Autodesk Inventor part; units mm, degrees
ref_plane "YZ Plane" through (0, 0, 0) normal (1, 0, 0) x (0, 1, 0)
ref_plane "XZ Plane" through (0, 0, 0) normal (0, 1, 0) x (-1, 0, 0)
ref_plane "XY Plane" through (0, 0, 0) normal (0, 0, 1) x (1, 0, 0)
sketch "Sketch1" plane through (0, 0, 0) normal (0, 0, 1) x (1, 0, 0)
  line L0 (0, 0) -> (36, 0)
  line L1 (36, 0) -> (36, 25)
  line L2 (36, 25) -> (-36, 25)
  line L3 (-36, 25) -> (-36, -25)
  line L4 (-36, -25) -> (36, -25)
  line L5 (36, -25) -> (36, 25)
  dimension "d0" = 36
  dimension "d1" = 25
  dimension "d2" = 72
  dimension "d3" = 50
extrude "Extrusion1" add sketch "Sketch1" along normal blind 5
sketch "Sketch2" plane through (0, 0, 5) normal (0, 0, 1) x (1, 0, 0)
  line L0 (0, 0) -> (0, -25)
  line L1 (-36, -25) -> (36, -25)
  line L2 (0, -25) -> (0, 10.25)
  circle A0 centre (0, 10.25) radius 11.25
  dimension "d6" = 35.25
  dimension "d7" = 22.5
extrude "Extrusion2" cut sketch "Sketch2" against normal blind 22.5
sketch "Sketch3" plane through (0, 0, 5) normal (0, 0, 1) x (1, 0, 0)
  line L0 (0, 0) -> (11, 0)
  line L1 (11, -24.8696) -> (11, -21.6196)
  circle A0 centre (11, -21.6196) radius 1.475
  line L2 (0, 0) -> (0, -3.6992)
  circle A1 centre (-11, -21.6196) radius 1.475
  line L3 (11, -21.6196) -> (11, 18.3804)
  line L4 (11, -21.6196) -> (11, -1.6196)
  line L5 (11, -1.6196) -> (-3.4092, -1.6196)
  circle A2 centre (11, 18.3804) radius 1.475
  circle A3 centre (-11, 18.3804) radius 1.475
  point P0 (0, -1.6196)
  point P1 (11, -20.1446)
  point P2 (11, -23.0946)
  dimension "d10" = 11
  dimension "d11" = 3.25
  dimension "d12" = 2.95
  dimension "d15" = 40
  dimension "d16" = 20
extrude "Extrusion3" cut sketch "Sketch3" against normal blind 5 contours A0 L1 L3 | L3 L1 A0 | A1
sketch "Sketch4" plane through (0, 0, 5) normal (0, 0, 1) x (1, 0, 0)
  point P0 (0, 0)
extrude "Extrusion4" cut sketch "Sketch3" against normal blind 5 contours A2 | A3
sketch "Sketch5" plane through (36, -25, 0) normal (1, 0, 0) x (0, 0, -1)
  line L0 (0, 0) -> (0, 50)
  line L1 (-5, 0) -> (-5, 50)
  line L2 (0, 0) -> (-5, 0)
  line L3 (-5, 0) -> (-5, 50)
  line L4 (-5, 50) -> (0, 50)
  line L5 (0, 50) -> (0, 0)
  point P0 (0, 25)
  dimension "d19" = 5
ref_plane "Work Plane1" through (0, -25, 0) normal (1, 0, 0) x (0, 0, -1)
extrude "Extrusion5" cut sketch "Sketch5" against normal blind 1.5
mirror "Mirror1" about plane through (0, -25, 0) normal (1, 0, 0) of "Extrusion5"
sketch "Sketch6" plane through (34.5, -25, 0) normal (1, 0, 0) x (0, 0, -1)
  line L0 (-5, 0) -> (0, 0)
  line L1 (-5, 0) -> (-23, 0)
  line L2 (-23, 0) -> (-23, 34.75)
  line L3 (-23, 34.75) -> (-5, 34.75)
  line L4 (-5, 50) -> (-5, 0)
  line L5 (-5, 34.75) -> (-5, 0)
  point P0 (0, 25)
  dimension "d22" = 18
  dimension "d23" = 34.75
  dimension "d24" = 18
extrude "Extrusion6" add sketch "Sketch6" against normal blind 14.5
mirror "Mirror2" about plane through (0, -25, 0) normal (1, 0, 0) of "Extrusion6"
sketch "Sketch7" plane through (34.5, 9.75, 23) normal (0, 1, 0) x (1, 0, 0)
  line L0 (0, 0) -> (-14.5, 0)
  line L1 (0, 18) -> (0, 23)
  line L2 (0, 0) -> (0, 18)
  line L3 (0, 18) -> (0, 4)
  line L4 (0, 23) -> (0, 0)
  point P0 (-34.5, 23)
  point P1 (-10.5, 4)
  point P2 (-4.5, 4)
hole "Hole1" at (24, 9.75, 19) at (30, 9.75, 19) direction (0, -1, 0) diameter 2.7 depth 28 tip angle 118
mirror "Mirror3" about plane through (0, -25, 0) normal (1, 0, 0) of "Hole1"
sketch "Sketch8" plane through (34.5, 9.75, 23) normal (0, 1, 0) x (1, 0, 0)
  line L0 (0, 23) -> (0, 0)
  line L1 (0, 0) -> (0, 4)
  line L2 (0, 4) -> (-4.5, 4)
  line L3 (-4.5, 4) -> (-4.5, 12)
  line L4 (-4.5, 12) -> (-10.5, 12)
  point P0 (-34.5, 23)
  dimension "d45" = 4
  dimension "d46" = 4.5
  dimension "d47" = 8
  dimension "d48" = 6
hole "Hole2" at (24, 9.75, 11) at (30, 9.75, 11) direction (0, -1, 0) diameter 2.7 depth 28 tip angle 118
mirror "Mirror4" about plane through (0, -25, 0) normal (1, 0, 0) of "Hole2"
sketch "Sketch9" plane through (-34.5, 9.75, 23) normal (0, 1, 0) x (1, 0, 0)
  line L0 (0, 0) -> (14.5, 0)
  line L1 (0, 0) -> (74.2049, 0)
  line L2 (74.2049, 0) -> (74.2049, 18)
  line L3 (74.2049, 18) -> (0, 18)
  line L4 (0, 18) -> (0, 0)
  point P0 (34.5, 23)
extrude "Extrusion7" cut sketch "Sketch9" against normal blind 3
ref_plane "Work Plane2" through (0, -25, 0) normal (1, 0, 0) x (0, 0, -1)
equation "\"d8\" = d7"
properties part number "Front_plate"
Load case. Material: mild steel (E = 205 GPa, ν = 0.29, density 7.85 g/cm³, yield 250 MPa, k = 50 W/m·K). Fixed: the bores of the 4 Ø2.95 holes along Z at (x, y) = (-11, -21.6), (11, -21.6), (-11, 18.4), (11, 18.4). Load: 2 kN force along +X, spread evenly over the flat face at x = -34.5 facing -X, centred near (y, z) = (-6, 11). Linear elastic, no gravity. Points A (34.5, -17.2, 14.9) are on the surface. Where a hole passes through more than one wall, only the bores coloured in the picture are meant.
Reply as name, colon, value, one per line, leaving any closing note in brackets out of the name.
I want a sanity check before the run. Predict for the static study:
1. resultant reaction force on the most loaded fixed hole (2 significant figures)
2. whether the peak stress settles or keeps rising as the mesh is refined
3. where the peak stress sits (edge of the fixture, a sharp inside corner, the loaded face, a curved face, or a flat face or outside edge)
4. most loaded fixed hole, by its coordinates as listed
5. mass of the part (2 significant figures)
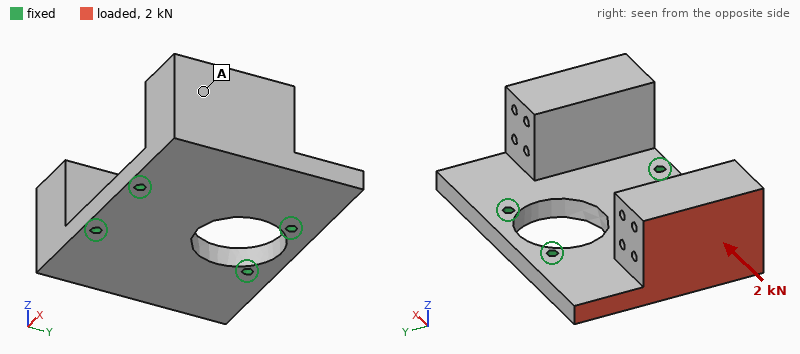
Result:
resultant reaction force on the most loaded fixed hole: 1000 N
whether the peak stress settles or keeps rising as the mesh is refined: keeps rising
where the peak stress sits: edge of the fixture
most loaded fixed hole, by its coordinates as listed: (-11, -21.6)
mass of the part: 240 g
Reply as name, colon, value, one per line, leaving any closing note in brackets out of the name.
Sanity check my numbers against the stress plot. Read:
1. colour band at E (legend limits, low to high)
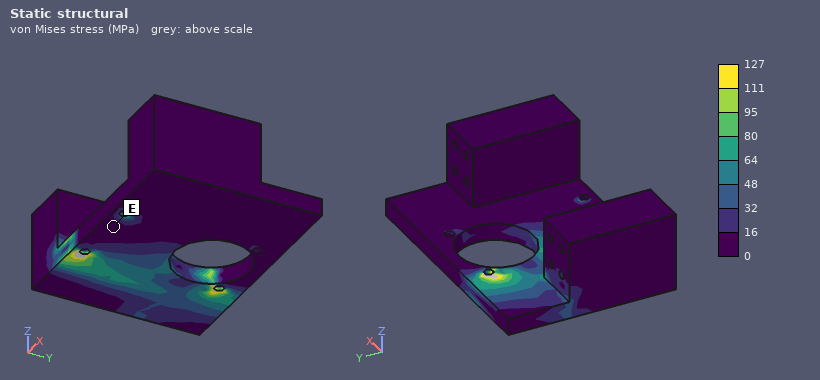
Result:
colour band at E: 0 to 16 MPa
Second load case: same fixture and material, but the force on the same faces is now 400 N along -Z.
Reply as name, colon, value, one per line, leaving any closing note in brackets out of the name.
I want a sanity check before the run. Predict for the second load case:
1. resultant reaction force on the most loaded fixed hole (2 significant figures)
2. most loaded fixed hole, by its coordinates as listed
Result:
resultant reaction force on the most loaded fixed hole: 340 N
most loaded fixed hole, by its coordinates as listed: (-11, -21.6)
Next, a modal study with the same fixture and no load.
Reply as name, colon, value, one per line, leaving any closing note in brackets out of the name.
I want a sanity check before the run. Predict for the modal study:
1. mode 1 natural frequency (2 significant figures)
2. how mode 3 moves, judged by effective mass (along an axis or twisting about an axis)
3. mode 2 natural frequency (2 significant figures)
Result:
mode 1 natural frequency: 2600 Hz
how mode 3 moves, judged by effective mass: along Y
mode 2 natural frequency: 2700 Hz
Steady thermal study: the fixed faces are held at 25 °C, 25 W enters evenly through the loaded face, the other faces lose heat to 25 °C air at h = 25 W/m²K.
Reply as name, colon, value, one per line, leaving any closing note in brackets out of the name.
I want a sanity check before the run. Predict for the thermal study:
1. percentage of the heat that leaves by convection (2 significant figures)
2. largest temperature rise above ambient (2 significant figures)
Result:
percentage of the heat that leaves by convection: 18 %
largest temperature rise above ambient: 49 K
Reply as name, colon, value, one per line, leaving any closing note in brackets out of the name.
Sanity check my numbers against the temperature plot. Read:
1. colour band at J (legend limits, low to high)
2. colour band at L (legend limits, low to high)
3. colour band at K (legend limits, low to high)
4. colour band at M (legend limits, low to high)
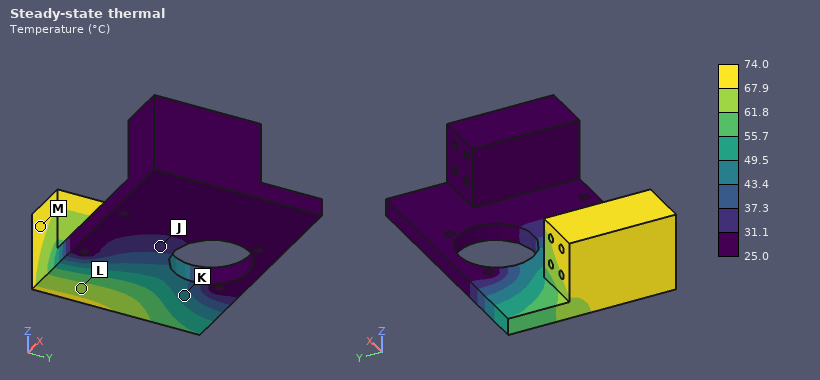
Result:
colour band at J: 31.1 to 37.3 °C
colour band at L: 61.8 to 67.9 °C
colour band at K: 43.4 to 49.5 °C
colour band at M: 67.9 to 74.0 °C
